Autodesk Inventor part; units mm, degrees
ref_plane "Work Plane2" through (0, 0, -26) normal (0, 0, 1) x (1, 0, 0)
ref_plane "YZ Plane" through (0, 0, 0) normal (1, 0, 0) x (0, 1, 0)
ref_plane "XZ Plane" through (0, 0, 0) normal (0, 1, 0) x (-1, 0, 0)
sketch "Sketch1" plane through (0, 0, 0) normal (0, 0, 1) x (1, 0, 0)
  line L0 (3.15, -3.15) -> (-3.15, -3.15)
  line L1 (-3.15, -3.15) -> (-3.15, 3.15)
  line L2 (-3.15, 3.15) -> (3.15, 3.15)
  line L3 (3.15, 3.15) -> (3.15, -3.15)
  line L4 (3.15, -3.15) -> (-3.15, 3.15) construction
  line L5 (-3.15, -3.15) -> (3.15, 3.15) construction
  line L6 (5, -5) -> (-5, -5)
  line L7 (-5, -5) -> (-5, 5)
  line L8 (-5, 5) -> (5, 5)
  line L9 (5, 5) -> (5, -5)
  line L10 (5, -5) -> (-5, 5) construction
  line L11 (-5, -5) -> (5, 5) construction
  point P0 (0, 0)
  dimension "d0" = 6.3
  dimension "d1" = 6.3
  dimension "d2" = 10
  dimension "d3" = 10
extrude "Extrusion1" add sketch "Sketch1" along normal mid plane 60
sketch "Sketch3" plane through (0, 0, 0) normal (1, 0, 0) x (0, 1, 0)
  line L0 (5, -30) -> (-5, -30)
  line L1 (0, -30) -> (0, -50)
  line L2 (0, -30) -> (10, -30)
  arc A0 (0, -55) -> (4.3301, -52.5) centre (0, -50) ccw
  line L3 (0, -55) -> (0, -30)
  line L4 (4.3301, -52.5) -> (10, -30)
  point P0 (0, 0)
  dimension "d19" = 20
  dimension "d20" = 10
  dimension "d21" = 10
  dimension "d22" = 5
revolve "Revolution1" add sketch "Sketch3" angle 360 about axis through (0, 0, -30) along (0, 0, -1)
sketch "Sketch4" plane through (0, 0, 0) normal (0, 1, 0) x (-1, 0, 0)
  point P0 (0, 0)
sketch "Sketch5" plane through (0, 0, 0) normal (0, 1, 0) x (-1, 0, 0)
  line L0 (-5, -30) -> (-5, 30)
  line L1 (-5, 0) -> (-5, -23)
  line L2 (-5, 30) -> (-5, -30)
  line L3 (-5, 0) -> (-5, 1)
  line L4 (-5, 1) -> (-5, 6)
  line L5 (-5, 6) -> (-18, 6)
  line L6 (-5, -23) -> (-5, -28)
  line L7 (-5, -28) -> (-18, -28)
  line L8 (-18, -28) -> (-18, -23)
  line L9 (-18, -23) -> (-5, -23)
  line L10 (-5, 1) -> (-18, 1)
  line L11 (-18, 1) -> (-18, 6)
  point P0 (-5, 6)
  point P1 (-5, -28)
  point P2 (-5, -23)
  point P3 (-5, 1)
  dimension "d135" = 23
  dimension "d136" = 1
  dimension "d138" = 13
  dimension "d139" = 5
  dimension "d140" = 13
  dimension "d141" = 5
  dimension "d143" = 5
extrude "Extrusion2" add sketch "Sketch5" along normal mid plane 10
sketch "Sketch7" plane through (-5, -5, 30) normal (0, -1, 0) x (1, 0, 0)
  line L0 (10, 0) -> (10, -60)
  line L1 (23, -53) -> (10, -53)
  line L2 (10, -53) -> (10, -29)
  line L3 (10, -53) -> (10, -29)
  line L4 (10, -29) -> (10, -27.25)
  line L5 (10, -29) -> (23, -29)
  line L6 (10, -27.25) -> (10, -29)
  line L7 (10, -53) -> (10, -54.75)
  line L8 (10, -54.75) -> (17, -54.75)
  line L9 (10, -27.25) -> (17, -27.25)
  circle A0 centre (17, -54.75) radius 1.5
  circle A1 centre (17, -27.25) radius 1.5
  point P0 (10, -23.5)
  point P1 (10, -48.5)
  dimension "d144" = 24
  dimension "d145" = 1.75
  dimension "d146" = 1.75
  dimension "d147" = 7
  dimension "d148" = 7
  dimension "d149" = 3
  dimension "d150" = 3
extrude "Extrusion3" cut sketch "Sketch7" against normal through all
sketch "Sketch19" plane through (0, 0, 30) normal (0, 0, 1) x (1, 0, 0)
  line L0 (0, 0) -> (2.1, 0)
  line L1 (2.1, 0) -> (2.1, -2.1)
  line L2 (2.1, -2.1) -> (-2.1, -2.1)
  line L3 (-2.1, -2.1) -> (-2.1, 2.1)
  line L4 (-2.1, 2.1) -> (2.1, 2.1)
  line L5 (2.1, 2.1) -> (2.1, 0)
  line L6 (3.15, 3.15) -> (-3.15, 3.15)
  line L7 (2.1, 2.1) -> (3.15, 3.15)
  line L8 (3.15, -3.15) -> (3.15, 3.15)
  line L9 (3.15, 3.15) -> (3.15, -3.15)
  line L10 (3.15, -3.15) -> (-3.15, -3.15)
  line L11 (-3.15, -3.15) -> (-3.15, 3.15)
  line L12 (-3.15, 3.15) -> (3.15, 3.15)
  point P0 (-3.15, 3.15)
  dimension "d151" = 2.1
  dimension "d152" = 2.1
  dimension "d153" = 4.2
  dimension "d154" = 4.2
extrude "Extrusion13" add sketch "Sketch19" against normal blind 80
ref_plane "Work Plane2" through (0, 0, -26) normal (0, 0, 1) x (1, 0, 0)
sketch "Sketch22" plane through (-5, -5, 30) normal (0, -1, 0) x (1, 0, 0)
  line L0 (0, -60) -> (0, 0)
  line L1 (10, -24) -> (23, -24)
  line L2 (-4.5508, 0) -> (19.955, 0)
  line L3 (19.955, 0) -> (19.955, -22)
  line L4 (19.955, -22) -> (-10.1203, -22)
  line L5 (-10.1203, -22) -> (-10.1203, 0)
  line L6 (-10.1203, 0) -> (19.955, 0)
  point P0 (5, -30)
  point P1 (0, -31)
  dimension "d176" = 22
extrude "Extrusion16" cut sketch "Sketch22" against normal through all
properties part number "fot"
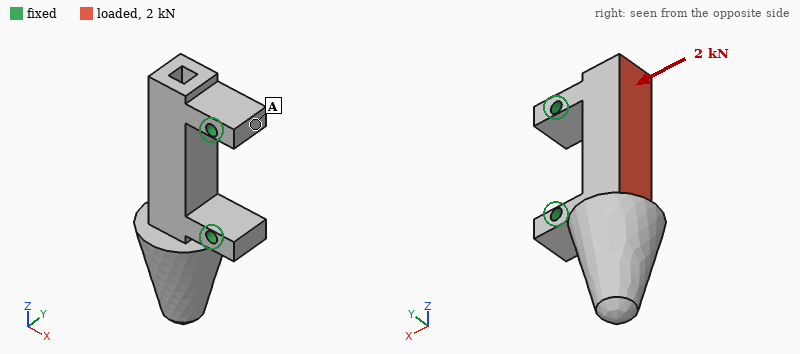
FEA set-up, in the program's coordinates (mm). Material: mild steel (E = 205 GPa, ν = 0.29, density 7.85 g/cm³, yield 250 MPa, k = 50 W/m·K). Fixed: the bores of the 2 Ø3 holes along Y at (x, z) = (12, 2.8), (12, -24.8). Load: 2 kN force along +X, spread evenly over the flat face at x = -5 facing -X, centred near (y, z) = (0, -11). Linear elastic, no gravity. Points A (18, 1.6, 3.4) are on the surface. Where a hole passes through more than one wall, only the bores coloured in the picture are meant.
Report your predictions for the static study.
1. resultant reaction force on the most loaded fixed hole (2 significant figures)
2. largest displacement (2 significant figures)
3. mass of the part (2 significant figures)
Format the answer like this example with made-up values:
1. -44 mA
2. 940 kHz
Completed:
1. 1.0 kN
2. 3.4 µm
3. 64 g
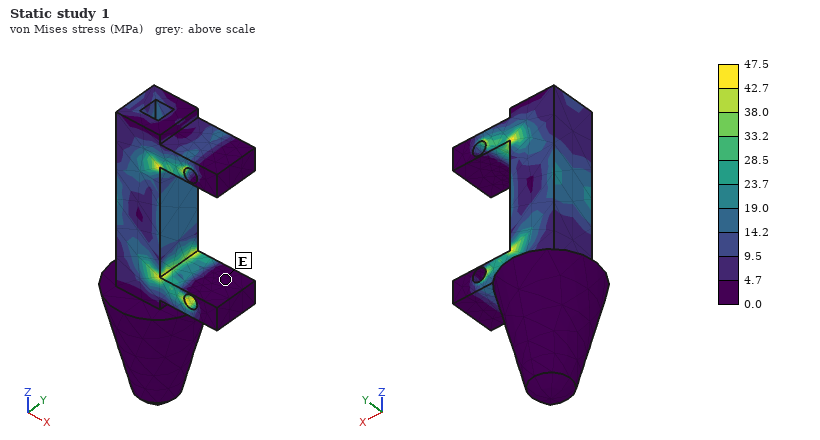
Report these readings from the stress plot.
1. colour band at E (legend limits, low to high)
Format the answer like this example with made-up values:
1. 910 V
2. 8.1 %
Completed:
1. 0.0 to 4.7 MPa
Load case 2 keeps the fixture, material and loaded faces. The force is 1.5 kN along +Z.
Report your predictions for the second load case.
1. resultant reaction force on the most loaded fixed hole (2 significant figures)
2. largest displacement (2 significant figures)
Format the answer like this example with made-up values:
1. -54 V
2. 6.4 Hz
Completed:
1. 970 N
2. 12 µm
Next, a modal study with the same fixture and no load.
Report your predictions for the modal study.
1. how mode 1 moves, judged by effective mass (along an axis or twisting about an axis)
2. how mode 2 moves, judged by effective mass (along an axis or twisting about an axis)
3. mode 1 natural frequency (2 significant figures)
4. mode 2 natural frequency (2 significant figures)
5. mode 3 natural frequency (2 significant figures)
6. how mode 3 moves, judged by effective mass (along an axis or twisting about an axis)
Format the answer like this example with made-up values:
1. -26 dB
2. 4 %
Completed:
1. along Y
2. along X
3. 5200 Hz
4. 6800 Hz
5. 11 kHz
6. along Y
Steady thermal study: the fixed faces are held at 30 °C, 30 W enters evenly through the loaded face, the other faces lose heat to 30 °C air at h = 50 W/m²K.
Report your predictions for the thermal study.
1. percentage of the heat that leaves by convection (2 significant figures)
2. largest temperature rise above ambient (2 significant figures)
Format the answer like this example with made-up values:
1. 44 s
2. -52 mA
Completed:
1. 23 %
2. 65 K
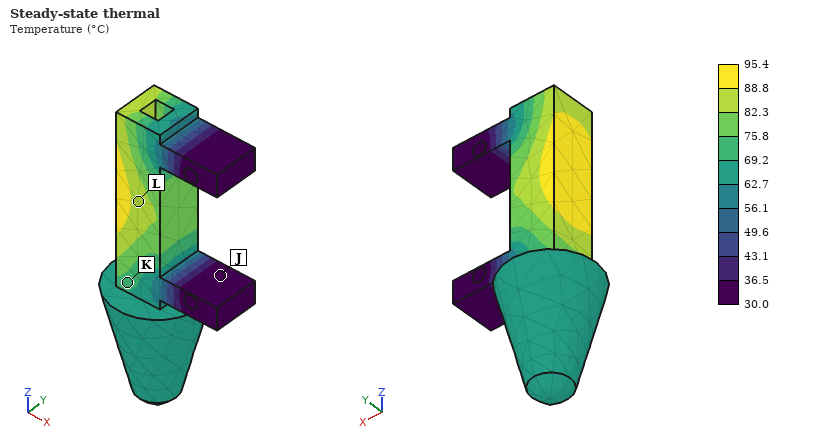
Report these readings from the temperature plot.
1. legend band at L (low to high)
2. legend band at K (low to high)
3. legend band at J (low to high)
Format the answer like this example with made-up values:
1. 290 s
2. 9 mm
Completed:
1. 82.3 to 88.8 °C
2. 69.2 to 75.8 °C
3. 30.0 to 36.5 °C
